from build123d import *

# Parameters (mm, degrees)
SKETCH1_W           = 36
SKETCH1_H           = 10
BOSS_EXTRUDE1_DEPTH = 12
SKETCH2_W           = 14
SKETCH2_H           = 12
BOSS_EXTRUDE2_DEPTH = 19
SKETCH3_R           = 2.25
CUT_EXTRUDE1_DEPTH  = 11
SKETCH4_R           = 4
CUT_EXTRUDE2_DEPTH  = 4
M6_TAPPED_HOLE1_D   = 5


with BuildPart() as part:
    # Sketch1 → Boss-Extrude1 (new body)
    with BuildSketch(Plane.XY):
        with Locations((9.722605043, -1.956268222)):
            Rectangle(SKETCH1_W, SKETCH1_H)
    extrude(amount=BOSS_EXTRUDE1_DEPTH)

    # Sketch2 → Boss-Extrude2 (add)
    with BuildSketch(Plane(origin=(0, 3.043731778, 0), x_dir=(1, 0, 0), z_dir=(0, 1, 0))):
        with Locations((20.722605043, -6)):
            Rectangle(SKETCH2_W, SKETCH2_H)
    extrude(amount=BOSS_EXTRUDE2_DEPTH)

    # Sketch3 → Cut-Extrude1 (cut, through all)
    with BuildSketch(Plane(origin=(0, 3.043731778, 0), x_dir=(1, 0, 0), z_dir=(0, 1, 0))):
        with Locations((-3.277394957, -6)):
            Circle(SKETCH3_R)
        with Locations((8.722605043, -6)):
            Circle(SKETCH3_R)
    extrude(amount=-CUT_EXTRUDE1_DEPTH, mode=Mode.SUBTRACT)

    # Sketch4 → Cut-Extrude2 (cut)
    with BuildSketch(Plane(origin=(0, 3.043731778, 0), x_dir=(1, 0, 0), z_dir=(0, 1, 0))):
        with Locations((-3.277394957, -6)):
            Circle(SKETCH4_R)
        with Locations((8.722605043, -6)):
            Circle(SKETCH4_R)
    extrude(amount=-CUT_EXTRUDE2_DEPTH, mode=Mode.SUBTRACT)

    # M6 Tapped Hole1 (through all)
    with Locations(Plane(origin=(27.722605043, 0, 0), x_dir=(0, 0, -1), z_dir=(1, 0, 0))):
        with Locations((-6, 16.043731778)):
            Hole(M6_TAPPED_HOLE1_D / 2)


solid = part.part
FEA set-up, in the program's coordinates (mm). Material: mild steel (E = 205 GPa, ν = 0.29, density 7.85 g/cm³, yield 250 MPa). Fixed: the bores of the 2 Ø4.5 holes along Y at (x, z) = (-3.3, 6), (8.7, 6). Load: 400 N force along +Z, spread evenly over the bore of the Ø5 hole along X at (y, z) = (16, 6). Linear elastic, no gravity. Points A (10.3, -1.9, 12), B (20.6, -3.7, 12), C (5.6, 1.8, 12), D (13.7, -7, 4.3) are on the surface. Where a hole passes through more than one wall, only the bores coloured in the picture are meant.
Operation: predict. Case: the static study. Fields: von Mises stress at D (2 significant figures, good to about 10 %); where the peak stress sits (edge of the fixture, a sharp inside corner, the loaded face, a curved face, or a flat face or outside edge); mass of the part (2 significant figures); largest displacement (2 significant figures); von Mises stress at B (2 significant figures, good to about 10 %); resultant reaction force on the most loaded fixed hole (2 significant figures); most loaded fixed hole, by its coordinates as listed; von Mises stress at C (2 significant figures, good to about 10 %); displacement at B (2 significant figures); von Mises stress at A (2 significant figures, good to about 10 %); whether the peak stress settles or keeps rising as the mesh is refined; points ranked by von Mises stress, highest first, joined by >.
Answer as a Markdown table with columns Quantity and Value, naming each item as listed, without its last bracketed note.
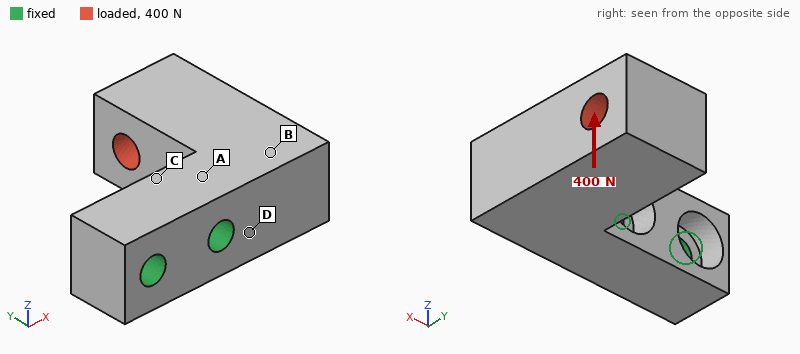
| Quantity | Value |
|---|---|
| von Mises stress at D | 32 MPa |
| where the peak stress sits | edge of the fixture |
| mass of the part | 52 g |
| largest displacement | 20 µm |
| von Mises stress at B | 8.7 MPa |
| resultant reaction force on the most loaded fixed hole | 550 N |
| most loaded fixed hole, by its coordinates as listed | (8.7, 6) |
| von Mises stress at C | 22 MPa |
| displacement at B | 3.8 µm |
| von Mises stress at A | 56 MPa |
| whether the peak stress settles or keeps rising as the mesh is refined | keeps rising |
| points ranked by von Mises stress, highest first, joined by > | A > D > C > B |
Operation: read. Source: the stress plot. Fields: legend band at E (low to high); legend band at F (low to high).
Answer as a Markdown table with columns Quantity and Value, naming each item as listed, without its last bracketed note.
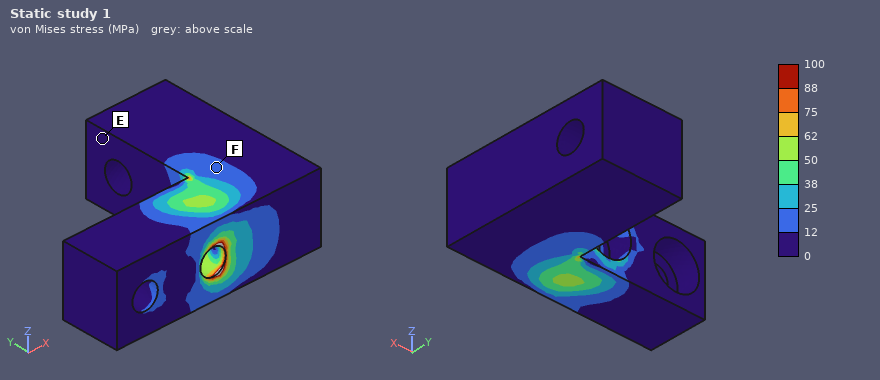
| Quantity | Value |
|---|---|
| legend band at E | 0 to 12 MPa |
| legend band at F | 12 to 25 MPa |
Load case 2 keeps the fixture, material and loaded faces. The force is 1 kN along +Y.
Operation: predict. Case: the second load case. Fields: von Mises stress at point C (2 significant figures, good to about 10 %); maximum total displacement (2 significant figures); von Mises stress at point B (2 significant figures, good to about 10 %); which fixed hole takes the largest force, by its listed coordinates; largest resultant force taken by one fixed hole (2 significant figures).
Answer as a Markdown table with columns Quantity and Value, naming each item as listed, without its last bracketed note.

| Quantity | Value |
|---|---|
| von Mises stress at point C | 37 MPa |
| maximum total displacement | 20 µm |
| von Mises stress at point B | 11 MPa |
| which fixed hole takes the largest force, by its listed coordinates | (8.7, 6) |
| largest resultant force taken by one fixed hole | 1.4 kN |
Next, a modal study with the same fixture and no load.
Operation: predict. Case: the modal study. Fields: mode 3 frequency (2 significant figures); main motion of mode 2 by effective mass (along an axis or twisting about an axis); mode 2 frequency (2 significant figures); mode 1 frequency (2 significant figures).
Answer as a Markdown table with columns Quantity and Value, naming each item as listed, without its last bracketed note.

| Quantity | Value |
|---|---|
| mode 3 frequency | 14 kHz |
| main motion of mode 2 by effective mass | along Z |
| mode 2 frequency | 6200 Hz |
| mode 1 frequency | 5800 Hz |
